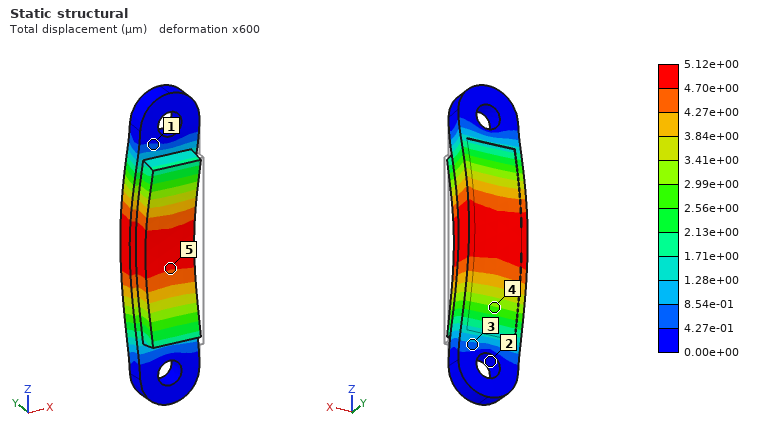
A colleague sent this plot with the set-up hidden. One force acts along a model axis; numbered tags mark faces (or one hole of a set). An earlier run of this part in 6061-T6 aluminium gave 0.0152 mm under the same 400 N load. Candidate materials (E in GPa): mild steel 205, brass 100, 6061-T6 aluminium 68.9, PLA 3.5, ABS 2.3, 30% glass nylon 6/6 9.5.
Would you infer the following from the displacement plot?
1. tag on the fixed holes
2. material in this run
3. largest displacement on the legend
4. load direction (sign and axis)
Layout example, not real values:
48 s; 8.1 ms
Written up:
2; mild steel; 5.12e+00 µm; +Y
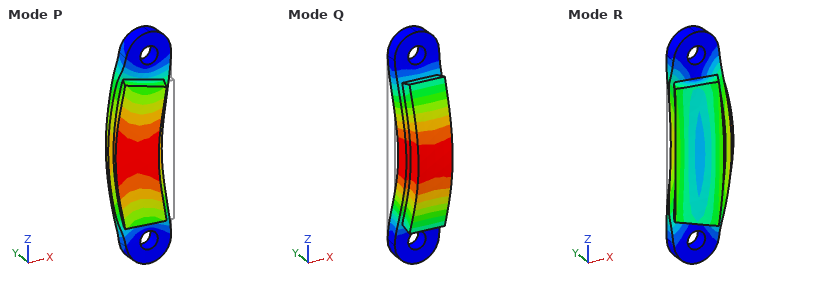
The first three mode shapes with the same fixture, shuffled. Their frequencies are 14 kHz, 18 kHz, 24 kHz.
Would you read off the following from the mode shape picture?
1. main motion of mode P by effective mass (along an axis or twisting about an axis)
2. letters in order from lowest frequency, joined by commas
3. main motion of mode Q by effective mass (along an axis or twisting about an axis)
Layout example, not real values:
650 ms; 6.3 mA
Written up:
along X; Q, P, R; along Y
